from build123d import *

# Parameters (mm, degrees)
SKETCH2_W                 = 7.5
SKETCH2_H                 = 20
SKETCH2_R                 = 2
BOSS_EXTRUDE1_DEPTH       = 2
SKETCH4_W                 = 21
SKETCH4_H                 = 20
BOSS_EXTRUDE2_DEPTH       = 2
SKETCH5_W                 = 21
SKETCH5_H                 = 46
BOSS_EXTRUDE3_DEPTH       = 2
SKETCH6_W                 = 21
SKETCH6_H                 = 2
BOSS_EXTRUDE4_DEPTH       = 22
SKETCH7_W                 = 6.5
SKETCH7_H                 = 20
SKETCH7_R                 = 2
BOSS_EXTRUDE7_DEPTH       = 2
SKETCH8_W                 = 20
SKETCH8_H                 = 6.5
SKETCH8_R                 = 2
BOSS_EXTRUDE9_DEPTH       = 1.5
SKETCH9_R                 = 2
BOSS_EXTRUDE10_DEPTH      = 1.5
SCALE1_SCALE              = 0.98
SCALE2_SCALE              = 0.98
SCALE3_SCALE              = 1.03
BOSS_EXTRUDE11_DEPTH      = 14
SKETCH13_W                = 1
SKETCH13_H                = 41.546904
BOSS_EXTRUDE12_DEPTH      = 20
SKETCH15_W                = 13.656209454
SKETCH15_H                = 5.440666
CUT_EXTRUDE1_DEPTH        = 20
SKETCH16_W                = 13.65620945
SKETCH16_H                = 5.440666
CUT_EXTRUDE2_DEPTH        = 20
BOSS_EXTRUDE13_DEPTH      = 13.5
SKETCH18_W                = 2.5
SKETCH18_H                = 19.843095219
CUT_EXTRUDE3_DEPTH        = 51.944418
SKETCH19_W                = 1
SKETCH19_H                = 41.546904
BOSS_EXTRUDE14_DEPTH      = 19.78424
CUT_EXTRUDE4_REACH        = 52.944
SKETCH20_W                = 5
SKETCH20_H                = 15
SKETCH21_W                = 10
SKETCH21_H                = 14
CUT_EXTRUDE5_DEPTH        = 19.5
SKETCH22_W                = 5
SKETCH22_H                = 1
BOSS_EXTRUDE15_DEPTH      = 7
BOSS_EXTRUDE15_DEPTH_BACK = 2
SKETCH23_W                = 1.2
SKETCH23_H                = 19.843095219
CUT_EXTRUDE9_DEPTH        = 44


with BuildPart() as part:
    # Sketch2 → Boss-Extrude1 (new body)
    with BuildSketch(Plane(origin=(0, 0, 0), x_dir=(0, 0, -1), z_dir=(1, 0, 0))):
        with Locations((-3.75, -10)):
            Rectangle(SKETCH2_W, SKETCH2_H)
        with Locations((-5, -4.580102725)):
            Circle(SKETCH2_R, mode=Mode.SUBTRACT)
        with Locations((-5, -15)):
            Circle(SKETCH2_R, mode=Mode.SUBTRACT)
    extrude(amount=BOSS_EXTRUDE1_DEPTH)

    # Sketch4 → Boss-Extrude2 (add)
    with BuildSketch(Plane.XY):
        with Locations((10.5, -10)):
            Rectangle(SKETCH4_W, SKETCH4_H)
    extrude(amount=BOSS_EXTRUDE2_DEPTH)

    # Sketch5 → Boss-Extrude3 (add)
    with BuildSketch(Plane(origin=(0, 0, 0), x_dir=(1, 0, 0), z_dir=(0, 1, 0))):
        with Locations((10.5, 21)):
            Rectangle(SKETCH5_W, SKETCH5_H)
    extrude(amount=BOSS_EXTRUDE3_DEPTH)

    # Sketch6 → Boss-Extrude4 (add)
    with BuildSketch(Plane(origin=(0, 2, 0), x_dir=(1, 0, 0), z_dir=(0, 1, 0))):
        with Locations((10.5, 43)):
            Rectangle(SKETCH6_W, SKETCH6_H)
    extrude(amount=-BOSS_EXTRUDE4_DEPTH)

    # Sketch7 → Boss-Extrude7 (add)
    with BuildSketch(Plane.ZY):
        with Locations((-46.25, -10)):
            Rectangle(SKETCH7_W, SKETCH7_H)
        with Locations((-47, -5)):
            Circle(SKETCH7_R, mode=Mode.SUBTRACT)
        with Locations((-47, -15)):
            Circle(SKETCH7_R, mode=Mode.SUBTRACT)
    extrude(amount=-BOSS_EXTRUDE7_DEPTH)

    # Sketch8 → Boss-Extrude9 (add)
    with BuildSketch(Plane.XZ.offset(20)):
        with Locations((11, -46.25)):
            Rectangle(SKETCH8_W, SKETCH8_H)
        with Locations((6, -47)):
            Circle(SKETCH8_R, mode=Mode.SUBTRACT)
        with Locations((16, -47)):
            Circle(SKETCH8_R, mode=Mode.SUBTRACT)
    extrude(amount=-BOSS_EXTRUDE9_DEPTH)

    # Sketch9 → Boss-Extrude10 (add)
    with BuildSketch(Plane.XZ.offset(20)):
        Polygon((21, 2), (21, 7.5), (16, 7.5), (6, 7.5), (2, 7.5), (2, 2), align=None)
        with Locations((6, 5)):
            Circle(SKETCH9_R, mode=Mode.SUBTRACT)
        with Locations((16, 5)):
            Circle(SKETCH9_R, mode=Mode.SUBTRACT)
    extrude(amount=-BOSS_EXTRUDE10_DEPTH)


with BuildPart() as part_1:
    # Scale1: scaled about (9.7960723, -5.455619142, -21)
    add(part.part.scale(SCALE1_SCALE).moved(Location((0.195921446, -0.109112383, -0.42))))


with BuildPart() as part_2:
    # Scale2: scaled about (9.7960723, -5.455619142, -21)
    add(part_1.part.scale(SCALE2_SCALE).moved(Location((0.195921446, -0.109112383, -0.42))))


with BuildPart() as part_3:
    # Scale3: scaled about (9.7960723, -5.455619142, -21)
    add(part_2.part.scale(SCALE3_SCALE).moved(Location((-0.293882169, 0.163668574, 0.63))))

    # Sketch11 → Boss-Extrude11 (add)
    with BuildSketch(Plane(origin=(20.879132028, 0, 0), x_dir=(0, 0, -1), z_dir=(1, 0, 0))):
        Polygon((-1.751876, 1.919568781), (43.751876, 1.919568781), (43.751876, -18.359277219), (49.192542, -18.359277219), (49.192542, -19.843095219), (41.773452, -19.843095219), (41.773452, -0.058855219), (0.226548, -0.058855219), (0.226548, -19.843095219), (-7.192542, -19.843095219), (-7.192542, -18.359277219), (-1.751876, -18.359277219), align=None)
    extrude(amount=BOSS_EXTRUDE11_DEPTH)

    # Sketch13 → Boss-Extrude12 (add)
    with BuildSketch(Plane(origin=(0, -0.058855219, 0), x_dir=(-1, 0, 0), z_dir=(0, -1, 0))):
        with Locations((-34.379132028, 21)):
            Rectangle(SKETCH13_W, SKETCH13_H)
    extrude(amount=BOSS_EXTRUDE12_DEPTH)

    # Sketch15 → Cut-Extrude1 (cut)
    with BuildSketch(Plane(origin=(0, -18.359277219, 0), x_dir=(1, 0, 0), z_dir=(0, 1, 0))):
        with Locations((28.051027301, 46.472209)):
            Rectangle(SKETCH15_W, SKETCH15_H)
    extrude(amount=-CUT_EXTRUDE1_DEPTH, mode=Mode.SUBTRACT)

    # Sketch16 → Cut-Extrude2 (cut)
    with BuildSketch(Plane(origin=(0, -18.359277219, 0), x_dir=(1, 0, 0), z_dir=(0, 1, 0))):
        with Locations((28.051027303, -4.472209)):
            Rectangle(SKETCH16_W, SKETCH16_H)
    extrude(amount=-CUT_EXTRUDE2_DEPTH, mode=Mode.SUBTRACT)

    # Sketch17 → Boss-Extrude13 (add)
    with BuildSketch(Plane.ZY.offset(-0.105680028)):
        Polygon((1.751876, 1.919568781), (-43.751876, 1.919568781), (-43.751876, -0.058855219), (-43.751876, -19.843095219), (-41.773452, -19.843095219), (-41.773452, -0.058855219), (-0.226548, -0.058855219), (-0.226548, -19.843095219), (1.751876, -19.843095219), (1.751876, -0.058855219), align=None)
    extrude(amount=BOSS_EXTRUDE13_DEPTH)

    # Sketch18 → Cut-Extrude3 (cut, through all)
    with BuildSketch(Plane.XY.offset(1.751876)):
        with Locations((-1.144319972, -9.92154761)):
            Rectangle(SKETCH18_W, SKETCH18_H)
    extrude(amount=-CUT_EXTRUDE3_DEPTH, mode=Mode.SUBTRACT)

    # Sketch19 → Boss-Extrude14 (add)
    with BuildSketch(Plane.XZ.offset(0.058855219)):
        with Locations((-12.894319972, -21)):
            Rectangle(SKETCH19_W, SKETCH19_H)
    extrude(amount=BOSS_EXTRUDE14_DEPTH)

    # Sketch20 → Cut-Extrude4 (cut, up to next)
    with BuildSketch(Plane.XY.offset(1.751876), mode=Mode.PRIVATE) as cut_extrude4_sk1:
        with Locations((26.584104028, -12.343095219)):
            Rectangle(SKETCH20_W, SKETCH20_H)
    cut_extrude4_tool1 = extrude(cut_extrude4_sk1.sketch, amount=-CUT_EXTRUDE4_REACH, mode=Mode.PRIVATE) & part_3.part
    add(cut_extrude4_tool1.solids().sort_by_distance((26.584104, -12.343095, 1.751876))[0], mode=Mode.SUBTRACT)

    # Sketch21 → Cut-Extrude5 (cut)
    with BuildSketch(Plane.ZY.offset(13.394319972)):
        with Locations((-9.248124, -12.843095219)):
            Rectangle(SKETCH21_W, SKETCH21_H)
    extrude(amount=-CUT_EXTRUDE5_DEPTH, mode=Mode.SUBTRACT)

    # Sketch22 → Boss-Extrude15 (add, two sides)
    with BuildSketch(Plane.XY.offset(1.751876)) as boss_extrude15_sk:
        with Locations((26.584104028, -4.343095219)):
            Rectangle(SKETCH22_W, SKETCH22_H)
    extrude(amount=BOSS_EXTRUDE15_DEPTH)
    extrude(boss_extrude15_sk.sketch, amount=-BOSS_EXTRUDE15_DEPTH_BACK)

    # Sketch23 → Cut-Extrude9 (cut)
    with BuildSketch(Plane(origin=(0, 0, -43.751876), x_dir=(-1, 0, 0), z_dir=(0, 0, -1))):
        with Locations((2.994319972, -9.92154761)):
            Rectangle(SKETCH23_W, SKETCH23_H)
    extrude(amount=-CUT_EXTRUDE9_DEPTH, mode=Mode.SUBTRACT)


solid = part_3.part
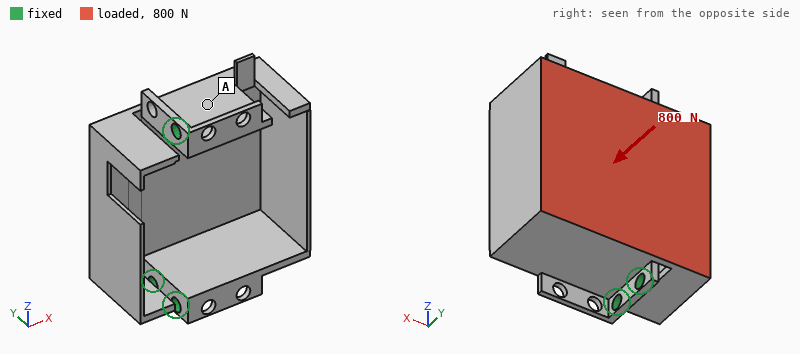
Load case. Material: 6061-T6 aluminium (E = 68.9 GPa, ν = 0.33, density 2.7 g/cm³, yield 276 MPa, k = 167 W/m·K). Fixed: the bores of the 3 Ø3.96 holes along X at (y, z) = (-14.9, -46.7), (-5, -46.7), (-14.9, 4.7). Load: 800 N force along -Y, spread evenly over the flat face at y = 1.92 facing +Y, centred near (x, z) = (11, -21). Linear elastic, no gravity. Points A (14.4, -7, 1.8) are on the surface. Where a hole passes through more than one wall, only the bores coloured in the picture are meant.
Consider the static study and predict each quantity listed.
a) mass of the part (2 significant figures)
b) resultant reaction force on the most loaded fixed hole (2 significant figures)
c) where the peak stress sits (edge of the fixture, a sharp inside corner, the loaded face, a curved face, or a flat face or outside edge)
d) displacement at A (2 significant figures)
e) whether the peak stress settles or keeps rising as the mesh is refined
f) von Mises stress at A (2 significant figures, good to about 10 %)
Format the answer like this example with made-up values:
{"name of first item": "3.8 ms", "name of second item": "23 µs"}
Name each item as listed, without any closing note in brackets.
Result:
{"mass of the part": "27 g", "resultant reaction force on the most loaded fixed hole": "450 N", "where the peak stress sits": "a sharp inside corner", "displacement at A": "0.081 mm", "whether the peak stress settles or keeps rising as the mesh is refined": "keeps rising", "von Mises stress at A": "18 MPa"}
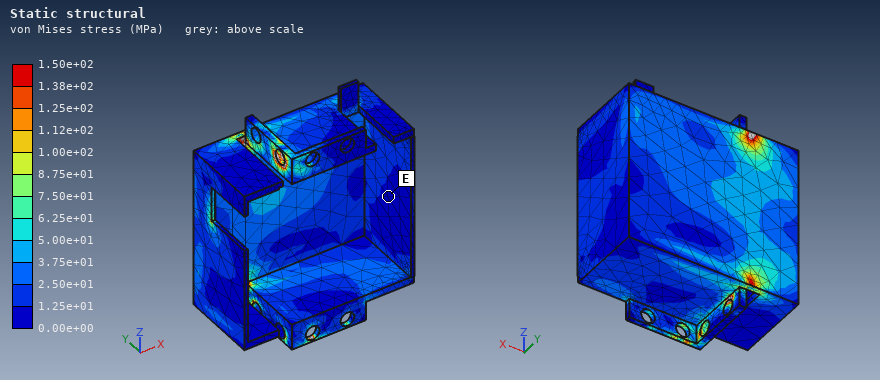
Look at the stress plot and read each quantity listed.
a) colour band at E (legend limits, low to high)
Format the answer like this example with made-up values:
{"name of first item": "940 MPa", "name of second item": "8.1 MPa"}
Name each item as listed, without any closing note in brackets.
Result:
{"colour band at E": "0.00e+00 to 1.25e+01 MPa"}
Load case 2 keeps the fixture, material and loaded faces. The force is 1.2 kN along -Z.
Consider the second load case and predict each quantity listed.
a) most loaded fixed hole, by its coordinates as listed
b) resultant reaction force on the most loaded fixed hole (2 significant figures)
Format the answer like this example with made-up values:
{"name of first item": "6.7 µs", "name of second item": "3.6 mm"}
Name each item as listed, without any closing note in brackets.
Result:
{"most loaded fixed hole, by its coordinates as listed": "(-5, -46.7)", "resultant reaction force on the most loaded fixed hole": "1.1 kN"}
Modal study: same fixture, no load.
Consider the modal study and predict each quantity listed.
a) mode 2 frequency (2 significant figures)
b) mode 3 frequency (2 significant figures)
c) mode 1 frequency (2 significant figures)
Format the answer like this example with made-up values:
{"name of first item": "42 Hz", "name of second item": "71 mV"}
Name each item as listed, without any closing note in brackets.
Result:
{"mode 2 frequency": "1700 Hz", "mode 3 frequency": "2300 Hz", "mode 1 frequency": "1600 Hz"}
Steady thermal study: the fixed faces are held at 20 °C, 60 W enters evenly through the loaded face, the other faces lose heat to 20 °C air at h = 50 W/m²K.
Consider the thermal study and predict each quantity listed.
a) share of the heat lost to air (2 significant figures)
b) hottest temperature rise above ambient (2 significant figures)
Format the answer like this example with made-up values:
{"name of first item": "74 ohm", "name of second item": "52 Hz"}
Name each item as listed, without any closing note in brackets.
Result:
{"share of the heat lost to air": "36 %", "hottest temperature rise above ambient": "60 K"}
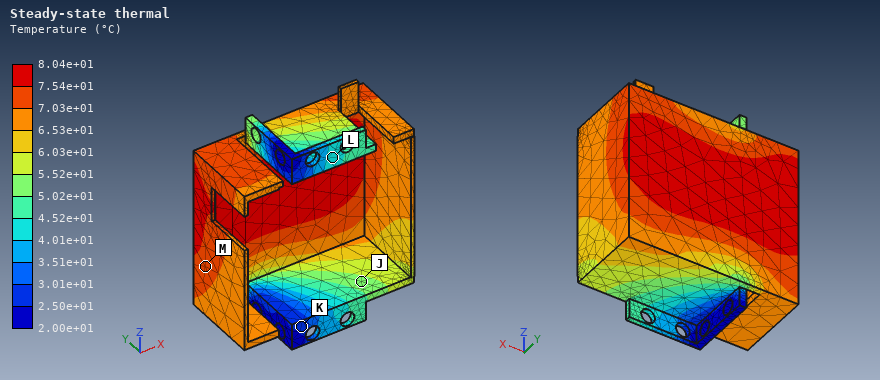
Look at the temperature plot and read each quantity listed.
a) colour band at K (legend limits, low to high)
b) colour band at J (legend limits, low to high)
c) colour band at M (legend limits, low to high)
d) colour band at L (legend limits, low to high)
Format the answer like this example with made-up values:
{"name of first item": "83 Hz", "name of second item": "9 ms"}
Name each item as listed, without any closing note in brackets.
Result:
{"colour band at K": "2.50e+01 to 3.01e+01 °C", "colour band at J": "5.02e+01 to 5.52e+01 °C", "colour band at M": "7.03e+01 to 7.54e+01 °C", "colour band at L": "4.01e+01 to 4.52e+01 °C"}
